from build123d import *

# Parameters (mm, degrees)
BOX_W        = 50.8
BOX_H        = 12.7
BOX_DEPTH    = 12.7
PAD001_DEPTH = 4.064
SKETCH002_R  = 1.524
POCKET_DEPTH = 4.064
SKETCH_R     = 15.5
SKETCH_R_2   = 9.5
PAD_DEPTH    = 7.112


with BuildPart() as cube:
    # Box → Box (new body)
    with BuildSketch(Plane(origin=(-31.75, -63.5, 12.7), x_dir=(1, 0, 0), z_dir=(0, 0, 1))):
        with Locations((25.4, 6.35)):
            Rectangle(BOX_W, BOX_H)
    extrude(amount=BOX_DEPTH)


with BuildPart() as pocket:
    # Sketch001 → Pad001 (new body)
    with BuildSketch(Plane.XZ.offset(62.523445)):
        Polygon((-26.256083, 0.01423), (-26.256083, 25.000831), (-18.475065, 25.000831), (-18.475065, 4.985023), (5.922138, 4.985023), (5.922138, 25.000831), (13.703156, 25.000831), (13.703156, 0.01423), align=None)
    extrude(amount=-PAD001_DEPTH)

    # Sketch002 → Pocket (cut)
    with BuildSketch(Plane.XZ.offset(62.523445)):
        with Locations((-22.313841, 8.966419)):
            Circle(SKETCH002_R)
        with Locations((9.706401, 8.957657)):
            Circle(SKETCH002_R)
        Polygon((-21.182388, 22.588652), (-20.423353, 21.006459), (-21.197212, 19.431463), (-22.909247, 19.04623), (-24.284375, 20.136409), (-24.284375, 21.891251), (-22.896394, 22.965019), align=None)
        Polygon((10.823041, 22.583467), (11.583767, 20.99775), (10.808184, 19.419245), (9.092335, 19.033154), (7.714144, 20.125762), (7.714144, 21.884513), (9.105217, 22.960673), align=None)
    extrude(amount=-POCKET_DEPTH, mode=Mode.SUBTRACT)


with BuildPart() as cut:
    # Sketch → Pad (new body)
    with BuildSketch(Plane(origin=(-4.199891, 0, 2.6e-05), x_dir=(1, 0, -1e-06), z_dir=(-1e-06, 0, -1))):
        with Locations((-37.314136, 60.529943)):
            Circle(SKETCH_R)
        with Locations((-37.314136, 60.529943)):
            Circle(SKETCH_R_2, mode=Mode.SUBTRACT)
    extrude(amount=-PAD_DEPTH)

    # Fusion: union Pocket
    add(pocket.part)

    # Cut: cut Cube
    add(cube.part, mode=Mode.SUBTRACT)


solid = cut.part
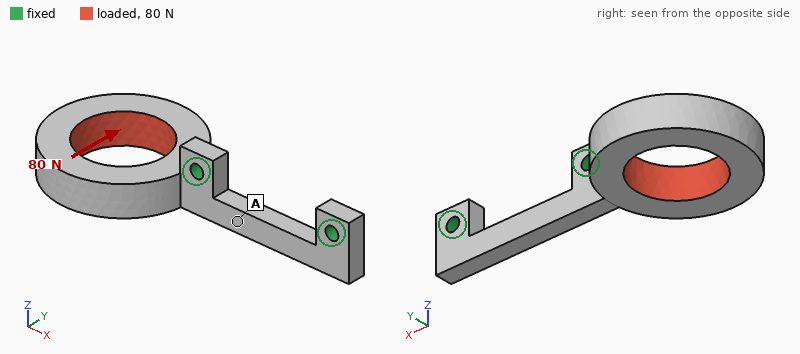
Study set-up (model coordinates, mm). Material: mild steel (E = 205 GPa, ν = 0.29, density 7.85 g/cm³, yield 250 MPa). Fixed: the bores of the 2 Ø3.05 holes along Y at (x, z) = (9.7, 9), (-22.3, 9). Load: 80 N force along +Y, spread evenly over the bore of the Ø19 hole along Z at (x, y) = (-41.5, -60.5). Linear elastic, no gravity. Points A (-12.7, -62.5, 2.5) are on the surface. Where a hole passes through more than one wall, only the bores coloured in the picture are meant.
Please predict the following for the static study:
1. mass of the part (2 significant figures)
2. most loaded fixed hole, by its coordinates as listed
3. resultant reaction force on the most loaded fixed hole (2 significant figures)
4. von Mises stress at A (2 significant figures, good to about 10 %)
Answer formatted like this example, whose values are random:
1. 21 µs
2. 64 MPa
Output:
1. 36 g
2. (-22.3, 9)
3. 90 N
4. 9.8 MPa
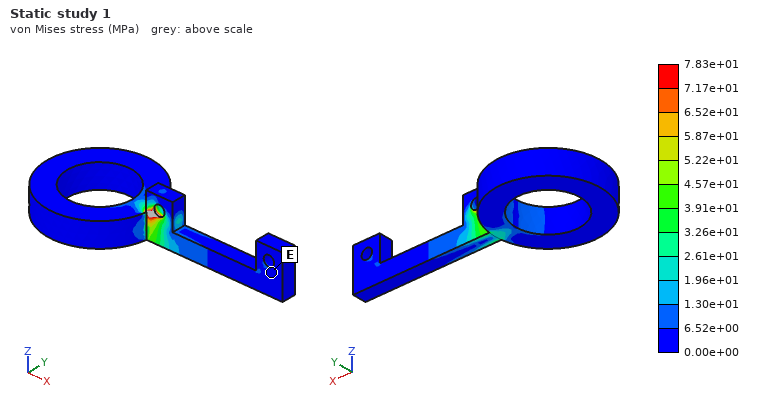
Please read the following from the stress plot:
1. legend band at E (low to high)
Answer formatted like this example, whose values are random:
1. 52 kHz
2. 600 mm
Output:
1. 0.00e+00 to 6.52e+00 MPa
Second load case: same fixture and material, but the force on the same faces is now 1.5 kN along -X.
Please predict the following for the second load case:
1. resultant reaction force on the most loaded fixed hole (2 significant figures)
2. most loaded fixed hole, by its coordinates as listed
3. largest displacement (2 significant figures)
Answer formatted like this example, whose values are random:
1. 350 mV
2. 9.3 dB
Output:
1. 1.1 kN
2. (-22.3, 9)
3. 33 µm
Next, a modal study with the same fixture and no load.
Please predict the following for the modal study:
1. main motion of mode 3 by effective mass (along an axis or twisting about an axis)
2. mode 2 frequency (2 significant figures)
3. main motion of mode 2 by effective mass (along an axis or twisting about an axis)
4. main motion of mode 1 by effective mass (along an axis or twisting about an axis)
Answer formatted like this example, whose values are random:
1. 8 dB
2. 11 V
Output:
1. twisting about X
2. 2500 Hz
3. along Z
4. along Y
